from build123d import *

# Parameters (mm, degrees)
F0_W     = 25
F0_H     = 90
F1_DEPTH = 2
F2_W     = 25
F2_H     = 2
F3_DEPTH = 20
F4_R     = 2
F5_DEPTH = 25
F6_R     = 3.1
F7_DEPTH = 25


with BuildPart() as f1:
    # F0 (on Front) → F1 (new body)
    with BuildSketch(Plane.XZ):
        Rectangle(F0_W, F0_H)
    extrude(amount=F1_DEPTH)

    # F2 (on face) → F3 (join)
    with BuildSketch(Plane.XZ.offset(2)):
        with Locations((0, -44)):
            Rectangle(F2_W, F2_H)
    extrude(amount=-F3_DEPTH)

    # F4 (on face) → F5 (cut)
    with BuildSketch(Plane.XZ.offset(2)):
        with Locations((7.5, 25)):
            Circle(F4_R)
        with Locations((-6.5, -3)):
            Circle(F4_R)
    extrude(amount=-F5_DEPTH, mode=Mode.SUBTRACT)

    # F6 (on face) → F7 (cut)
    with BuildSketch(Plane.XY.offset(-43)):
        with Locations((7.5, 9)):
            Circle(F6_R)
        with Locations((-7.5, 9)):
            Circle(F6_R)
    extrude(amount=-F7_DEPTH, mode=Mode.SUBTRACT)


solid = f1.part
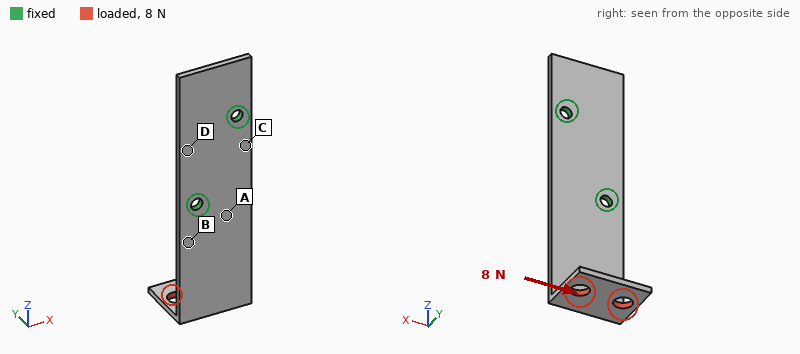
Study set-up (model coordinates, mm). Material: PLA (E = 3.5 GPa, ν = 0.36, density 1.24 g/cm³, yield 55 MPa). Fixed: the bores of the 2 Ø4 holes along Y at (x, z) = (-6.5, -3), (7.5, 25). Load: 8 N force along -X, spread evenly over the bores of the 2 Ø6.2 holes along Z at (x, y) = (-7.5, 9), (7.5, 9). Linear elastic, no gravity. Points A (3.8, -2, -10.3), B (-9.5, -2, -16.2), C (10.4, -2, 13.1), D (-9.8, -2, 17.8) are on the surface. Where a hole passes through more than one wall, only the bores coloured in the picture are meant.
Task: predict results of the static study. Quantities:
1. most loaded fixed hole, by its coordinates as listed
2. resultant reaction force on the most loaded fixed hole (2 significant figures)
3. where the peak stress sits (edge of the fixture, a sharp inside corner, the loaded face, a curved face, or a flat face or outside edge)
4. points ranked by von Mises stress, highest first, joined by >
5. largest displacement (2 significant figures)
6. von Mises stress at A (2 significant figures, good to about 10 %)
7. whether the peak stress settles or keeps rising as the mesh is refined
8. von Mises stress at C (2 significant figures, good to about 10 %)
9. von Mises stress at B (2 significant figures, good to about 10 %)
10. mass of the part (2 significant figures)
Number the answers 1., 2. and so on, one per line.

1. (-6.5, -3)
2. 17 N
3. edge of the fixture
4. B > A > C > D
5. 0.95 mm
6. 2.7 MPa
7. keeps rising
8. 1.8 MPa
9. 4.7 MPa
10. 6.5 g
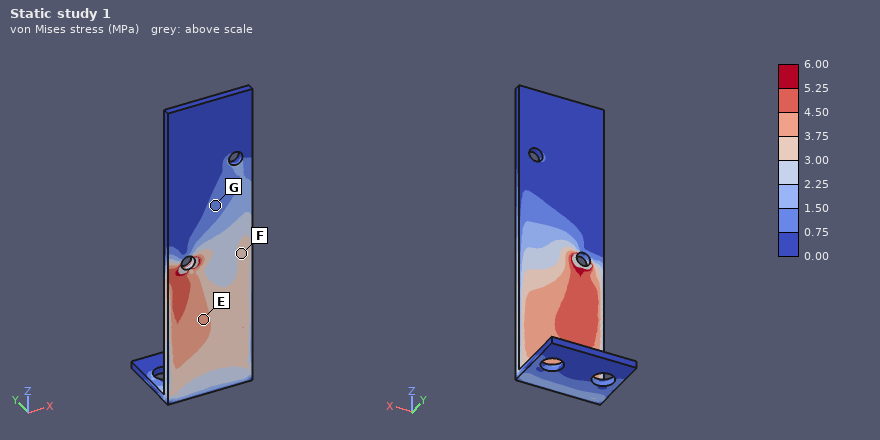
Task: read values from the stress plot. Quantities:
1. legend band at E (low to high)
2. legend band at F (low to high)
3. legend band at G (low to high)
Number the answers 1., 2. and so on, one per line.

1. 3.75 to 4.50 MPa
2. 3.00 to 3.75 MPa
3. 0.75 to 1.50 MPa
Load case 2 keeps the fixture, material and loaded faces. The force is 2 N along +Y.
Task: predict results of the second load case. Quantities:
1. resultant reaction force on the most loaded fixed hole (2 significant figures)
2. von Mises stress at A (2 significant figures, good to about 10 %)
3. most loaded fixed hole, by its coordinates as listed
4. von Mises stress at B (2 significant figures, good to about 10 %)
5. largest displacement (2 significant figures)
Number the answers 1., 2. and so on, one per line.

1. 2.9 N
2. 3.4 MPa
3. (-6.5, -3)
4. 3.6 MPa
5. 1.0 mm
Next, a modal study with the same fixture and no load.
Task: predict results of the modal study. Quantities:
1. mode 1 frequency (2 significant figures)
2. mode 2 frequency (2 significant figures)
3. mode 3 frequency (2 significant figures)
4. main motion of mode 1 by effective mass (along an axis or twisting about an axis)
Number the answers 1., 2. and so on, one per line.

1. 190 Hz
2. 480 Hz
3. 820 Hz
4. along Y
